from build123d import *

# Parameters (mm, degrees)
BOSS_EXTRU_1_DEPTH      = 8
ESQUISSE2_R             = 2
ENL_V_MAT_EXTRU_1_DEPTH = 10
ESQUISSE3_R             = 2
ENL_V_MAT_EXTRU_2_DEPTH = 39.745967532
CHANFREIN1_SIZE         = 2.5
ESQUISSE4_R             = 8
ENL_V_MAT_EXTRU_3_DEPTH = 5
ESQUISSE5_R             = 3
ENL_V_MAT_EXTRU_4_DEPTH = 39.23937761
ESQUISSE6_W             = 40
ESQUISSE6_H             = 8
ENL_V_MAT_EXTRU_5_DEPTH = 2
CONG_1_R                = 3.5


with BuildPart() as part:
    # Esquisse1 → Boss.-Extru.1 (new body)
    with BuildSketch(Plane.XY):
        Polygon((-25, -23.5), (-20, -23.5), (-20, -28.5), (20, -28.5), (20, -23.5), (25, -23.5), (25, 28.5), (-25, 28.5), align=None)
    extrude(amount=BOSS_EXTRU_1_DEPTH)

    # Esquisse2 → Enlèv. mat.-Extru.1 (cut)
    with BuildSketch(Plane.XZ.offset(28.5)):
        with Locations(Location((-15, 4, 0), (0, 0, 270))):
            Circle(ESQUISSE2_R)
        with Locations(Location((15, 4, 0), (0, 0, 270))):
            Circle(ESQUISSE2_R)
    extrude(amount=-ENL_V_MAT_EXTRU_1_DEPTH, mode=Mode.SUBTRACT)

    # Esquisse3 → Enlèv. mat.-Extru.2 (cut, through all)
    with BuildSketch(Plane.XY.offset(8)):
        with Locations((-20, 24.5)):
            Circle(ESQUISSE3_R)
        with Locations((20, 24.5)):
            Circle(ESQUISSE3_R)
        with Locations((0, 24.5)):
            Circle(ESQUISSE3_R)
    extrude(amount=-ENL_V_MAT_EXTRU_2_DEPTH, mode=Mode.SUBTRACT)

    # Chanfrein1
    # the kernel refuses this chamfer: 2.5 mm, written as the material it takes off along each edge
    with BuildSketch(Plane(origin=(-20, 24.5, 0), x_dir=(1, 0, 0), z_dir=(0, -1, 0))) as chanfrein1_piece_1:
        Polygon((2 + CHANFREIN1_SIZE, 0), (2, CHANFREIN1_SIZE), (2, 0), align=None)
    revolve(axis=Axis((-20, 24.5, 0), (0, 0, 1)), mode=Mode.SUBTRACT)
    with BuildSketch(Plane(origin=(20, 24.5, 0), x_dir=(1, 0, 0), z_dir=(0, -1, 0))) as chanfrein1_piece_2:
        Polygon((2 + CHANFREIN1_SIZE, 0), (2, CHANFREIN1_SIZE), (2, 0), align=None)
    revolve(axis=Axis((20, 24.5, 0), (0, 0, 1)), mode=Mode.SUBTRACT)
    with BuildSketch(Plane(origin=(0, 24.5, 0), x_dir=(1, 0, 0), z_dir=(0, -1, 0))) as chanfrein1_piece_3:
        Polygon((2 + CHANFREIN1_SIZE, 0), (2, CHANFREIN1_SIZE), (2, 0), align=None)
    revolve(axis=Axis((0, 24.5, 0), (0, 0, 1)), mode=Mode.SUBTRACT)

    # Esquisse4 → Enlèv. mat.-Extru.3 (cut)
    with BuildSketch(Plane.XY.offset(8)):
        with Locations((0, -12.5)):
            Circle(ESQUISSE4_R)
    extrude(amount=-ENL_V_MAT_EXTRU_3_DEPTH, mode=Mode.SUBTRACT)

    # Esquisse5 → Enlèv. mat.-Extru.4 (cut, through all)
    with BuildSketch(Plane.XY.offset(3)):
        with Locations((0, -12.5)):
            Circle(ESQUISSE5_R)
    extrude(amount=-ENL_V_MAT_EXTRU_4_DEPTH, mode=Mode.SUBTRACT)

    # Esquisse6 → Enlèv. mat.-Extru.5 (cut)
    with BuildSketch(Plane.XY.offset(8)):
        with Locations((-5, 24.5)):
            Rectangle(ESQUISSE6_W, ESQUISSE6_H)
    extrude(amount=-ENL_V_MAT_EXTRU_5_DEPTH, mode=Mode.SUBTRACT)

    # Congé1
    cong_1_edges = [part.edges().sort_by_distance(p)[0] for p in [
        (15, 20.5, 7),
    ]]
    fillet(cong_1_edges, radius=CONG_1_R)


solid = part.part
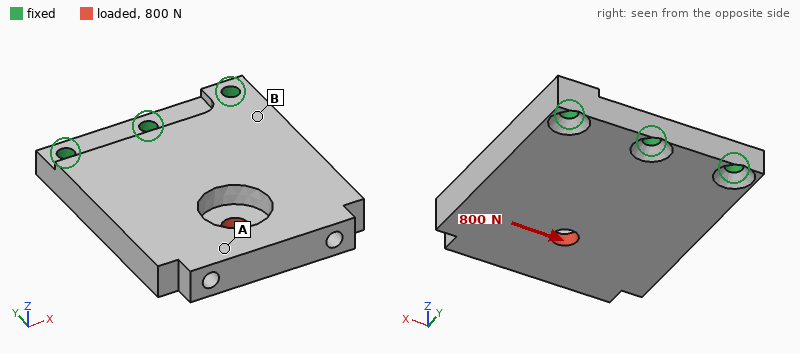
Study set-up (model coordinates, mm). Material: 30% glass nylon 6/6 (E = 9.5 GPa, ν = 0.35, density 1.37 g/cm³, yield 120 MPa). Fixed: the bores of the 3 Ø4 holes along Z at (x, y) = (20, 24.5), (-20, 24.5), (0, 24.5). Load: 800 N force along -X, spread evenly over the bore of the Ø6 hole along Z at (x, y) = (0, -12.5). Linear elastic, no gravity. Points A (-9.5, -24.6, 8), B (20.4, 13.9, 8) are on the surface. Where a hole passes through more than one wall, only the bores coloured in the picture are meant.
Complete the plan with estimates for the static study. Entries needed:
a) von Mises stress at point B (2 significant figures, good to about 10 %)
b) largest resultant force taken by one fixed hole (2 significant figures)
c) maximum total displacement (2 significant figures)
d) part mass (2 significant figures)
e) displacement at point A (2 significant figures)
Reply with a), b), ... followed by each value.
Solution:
a) 7.2 MPa
b) 780 N
c) 0.11 mm
d) 27 g
e) 0.080 mm
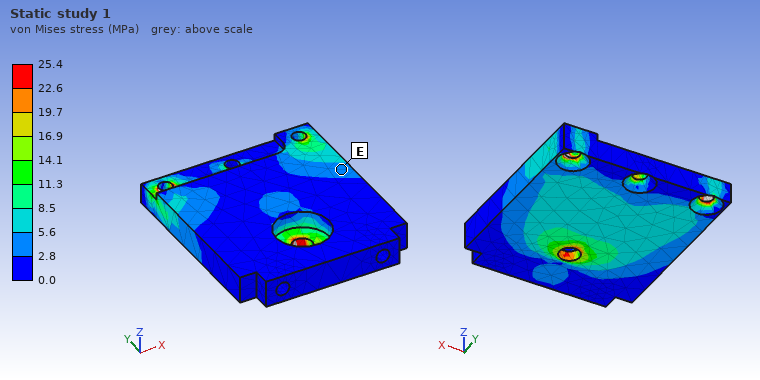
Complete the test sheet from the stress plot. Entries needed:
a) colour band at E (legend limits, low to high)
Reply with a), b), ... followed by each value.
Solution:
a) 2.8 to 5.6 MPa
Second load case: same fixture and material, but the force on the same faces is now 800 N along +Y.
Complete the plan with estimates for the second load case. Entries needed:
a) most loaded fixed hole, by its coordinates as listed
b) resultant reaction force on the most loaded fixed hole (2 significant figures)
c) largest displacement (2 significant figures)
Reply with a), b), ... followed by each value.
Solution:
a) (0, 24.5)
b) 310 N
c) 0.20 mm
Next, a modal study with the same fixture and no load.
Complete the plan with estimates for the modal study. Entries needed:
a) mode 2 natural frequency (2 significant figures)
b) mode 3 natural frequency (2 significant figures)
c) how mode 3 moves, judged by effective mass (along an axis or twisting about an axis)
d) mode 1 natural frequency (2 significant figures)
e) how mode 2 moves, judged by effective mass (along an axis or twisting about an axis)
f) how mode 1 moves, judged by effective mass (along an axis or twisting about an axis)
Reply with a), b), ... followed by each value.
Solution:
a) 2700 Hz
b) 4800 Hz
c) along X
d) 920 Hz
e) twisting about Y
f) along Z
